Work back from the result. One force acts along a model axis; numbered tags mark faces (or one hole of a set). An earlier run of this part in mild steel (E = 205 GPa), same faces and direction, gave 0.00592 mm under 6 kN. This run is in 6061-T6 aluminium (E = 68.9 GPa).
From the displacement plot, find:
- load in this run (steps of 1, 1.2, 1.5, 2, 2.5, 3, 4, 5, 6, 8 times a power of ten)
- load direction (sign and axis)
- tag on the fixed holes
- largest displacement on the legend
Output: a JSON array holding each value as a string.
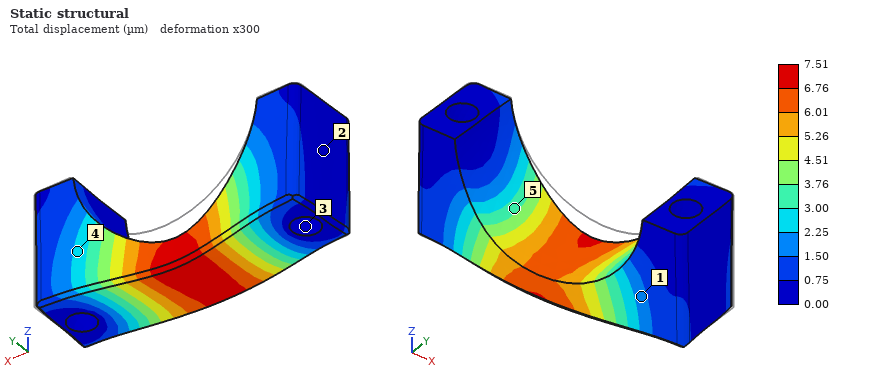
["2.5 kN", "-Y", "3", "7.51 µm"]
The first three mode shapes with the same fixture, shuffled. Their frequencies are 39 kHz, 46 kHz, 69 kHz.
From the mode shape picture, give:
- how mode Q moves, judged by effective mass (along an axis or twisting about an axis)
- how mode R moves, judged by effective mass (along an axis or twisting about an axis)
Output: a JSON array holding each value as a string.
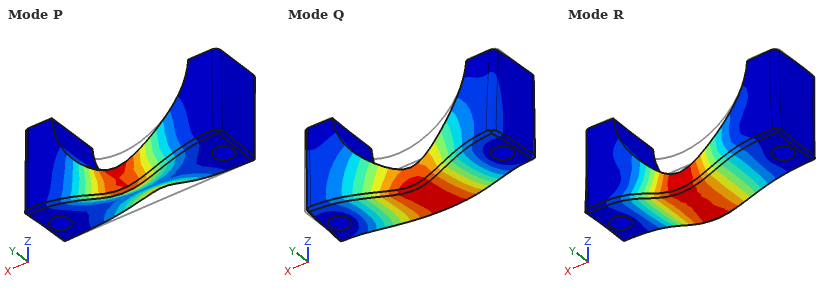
["along Y", "along Z"]
